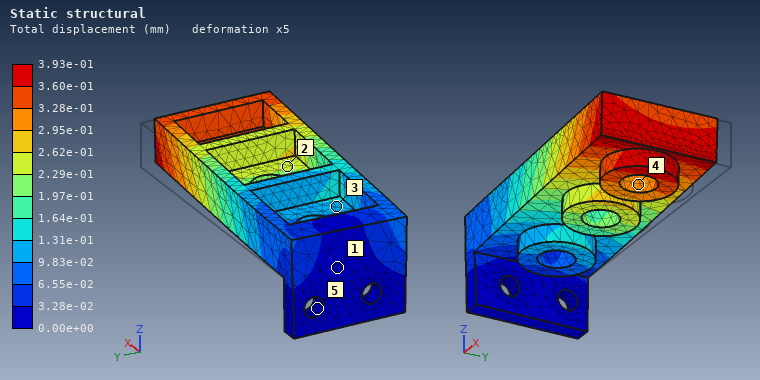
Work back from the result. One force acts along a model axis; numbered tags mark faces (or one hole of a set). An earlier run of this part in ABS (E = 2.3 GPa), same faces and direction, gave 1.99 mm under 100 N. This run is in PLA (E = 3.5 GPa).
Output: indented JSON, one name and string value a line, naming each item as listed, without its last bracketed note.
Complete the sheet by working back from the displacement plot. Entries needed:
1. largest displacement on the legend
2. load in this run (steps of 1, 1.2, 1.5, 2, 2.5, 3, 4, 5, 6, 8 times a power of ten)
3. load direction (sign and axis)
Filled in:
{
  "largest displacement on the legend": "3.93e-01 mm",
  "load in this run": "30 N",
  "load direction": "-Y"
}
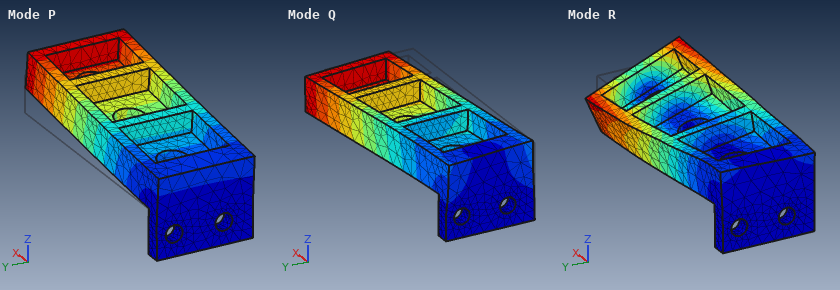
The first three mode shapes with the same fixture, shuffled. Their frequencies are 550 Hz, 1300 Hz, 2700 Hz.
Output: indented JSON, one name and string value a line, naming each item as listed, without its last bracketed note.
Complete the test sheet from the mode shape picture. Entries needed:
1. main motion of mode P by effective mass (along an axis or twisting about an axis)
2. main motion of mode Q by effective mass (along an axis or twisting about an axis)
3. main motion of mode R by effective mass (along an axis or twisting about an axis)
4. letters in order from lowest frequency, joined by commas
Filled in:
{
  "main motion of mode P by effective mass": "along Z",
  "main motion of mode Q by effective mass": "along Y",
  "main motion of mode R by effective mass": "twisting about X",
  "letters in order from lowest frequency, joined by commas": "P, Q, R"
}
